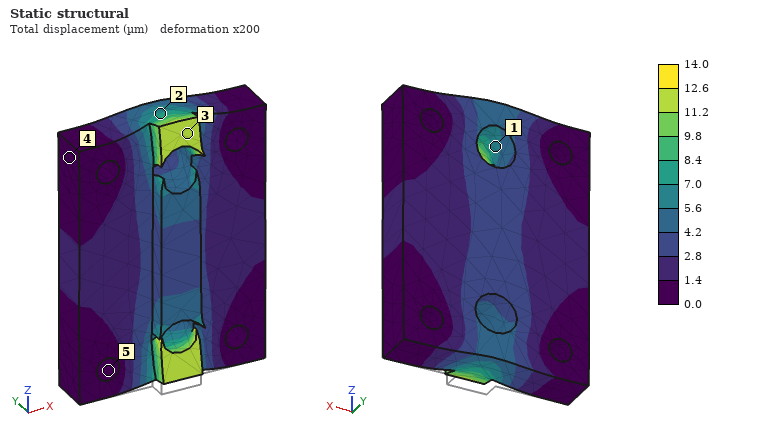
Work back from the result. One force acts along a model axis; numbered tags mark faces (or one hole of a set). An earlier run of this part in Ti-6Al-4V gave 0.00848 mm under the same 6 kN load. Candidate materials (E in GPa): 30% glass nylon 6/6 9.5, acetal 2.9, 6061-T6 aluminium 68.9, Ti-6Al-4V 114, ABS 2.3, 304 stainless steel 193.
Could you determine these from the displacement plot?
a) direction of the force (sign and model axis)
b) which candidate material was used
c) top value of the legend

+Z
6061-T6 aluminium
14.0 µm
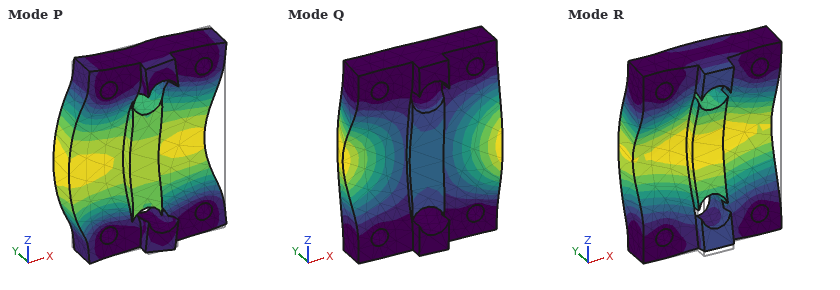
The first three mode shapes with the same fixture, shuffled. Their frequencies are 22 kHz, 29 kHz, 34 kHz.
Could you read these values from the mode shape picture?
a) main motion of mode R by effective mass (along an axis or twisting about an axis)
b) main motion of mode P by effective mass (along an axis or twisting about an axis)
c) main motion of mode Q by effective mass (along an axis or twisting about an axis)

along Y
along X
twisting about Z
